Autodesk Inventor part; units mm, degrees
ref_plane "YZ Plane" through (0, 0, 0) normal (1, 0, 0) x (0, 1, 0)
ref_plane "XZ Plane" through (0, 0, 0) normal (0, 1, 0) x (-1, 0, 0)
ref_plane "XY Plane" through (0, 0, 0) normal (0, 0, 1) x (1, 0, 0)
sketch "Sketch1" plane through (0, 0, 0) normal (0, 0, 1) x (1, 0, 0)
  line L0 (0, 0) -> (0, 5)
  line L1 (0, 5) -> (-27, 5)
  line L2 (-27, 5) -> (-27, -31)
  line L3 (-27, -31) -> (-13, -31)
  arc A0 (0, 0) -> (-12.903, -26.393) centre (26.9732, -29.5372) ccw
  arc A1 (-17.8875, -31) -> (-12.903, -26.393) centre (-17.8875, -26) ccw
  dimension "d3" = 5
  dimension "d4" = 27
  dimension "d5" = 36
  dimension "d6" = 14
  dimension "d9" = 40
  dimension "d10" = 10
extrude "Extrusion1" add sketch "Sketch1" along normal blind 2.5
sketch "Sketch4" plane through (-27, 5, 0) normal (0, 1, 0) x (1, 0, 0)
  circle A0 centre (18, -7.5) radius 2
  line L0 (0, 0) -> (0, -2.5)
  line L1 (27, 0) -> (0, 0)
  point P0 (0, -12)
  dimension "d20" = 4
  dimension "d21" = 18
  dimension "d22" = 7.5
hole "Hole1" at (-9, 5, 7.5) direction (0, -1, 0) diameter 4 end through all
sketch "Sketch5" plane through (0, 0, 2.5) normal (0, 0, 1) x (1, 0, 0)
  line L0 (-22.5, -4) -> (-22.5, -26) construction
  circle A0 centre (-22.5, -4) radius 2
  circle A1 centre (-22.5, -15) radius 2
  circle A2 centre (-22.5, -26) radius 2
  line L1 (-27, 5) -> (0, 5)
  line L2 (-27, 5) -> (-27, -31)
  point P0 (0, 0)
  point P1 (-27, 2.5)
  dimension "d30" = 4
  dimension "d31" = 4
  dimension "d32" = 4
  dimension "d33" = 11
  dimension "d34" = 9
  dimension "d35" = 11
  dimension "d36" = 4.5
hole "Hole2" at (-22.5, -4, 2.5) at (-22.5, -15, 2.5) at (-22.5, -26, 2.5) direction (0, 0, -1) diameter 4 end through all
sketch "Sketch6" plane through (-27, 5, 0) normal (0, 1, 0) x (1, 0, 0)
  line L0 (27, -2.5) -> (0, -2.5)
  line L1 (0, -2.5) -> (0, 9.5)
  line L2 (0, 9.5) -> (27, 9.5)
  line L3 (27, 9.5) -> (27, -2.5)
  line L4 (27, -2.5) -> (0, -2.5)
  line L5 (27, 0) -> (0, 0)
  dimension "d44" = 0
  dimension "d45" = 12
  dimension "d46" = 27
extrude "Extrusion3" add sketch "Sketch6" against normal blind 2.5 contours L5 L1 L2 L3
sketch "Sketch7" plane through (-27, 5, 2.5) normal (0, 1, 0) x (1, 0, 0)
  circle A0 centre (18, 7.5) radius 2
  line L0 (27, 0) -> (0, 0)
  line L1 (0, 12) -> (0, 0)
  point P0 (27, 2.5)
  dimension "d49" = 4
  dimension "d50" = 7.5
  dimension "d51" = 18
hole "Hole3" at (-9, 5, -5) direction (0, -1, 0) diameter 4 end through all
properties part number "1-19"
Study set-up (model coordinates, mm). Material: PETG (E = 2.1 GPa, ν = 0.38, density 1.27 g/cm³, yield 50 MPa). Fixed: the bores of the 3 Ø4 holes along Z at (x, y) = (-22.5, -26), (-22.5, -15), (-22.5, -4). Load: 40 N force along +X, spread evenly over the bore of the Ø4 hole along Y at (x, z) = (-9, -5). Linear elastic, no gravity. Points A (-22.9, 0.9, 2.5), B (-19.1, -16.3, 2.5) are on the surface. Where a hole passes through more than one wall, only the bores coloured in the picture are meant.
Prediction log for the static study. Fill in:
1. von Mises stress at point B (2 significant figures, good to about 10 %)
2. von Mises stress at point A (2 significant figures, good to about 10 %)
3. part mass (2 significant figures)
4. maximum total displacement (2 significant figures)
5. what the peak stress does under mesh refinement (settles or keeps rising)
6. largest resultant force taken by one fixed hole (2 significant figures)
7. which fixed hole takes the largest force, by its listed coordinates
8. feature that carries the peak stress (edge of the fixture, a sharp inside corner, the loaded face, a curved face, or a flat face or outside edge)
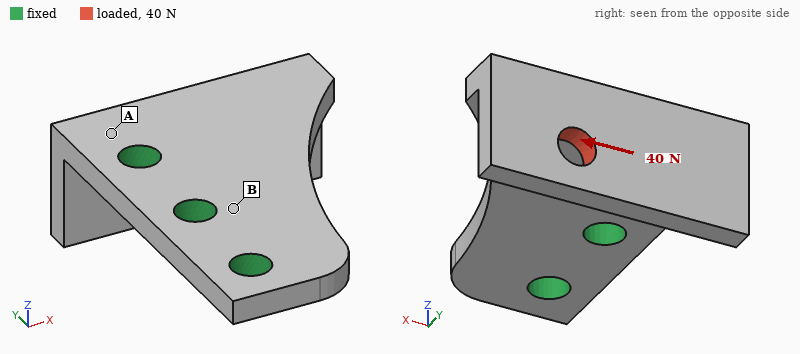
2.3 MPa
6.4 MPa
2.8 g
0.52 mm
keeps rising
52 N
(-22.5, -4)
edge of the fixture
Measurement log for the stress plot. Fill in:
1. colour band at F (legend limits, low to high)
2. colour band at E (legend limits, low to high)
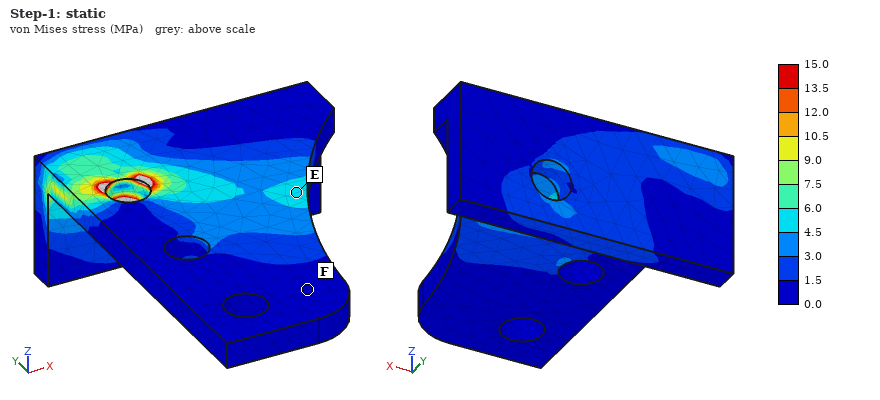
0.0 to 1.5 MPa
4.5 to 6.0 MPa
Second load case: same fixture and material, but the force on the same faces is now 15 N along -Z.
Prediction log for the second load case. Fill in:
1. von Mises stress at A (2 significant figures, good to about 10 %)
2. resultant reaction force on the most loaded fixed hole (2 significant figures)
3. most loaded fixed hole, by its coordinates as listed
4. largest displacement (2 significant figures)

6.9 MPa
19 N
(-22.5, -4)
0.46 mm
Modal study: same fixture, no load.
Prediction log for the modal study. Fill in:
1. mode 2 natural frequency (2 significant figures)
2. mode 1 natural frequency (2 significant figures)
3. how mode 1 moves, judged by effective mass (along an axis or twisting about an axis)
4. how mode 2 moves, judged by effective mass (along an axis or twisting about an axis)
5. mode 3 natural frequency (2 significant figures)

2100 Hz
1100 Hz
along Z
along Y
3600 Hz
